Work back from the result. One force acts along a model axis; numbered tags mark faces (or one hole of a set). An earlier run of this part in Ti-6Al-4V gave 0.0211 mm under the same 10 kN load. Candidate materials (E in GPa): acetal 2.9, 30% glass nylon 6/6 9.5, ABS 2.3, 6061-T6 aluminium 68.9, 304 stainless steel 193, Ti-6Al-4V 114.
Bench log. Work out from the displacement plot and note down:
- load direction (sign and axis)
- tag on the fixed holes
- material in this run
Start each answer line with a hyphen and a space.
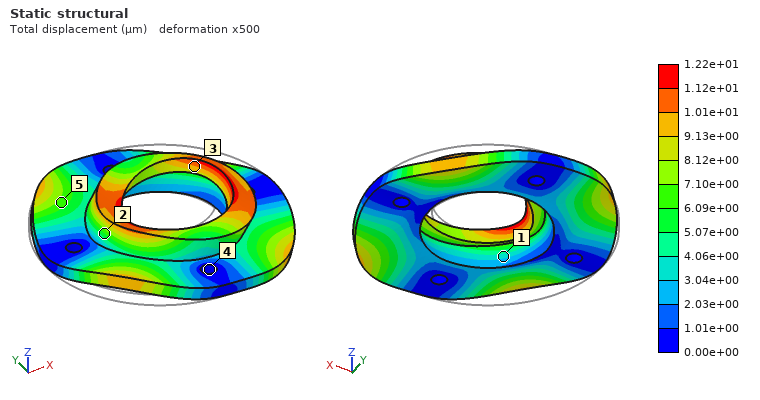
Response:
- +X
- 4
- 304 stainless steel
